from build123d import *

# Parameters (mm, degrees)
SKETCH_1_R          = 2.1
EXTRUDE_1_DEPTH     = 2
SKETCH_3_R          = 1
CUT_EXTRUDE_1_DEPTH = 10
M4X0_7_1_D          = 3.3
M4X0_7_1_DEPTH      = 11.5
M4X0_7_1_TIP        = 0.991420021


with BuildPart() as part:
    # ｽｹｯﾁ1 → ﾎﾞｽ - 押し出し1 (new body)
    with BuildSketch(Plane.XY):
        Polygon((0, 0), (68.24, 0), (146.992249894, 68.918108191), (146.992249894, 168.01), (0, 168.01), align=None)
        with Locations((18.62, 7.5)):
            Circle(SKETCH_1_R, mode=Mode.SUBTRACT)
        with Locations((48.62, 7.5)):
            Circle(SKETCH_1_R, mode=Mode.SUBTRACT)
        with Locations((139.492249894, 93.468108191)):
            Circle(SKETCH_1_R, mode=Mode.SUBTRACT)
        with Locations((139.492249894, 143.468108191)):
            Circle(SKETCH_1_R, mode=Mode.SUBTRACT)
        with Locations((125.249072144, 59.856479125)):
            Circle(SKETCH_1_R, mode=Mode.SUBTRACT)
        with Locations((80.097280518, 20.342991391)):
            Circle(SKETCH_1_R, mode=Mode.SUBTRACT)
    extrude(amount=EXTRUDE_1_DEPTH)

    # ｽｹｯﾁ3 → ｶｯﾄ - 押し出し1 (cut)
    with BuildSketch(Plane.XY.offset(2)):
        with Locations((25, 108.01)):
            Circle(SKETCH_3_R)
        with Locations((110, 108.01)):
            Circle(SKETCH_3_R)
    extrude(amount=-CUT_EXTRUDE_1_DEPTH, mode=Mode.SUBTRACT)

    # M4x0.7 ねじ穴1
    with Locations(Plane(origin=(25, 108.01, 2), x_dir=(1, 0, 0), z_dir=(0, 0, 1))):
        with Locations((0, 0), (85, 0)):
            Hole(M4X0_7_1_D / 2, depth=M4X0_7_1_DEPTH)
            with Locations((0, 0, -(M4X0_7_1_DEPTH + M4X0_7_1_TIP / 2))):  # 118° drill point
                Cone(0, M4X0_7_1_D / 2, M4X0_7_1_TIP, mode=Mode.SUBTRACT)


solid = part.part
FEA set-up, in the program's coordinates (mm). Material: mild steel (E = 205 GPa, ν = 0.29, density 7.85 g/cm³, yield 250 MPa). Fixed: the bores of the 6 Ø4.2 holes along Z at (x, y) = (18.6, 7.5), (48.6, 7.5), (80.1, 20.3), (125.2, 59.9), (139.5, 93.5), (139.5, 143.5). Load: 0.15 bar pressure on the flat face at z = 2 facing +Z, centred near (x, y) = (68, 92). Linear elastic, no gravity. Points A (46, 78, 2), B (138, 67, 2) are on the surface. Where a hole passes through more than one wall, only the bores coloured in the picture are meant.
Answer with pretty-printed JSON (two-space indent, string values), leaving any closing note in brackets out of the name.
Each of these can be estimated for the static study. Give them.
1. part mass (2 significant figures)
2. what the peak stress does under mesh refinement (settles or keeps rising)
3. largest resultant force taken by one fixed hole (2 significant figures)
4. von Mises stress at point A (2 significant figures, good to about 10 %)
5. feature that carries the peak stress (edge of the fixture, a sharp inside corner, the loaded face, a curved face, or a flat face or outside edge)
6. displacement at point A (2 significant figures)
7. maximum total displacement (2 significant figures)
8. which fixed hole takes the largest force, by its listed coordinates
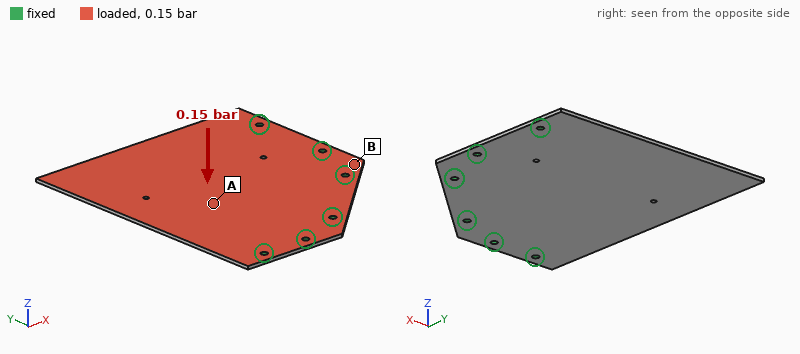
{
  "part mass": "340 g",
  "what the peak stress does under mesh refinement": "keeps rising",
  "largest resultant force taken by one fixed hole": "120 N",
  "von Mises stress at point A": "38 MPa",
  "feature that carries the peak stress": "edge of the fixture",
  "displacement at point A": "0.56 mm",
  "maximum total displacement": "2.3 mm",
  "which fixed hole takes the largest force, by its listed coordinates": "(139.5, 143.5)"
}
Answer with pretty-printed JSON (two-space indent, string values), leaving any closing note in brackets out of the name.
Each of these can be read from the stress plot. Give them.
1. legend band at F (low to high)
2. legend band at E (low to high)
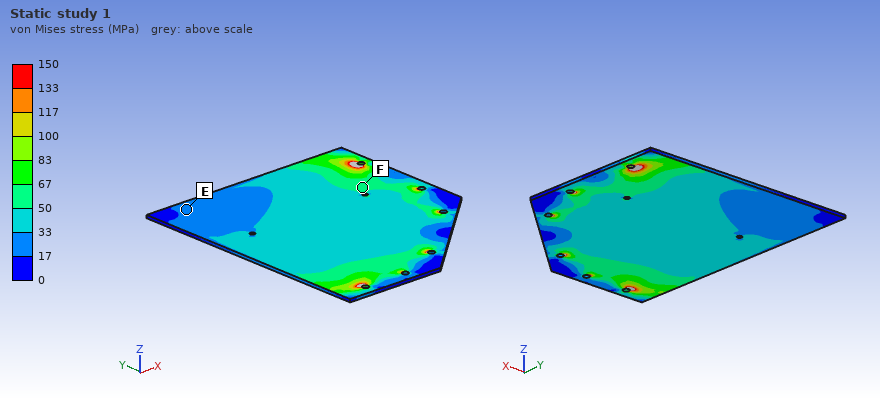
{
  "legend band at F": "50 to 67 MPa",
  "legend band at E": "17 to 33 MPa"
}
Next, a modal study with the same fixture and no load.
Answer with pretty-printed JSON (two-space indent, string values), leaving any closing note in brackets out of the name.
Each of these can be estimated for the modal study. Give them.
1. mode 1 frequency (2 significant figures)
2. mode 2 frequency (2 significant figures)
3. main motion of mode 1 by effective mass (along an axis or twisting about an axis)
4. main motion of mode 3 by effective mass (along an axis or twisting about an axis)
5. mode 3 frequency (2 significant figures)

{
  "mode 1 frequency": "150 Hz",
  "mode 2 frequency": "480 Hz",
  "main motion of mode 1 by effective mass": "along Z",
  "main motion of mode 3 by effective mass": "along Z",
  "mode 3 frequency": "610 Hz"
}
